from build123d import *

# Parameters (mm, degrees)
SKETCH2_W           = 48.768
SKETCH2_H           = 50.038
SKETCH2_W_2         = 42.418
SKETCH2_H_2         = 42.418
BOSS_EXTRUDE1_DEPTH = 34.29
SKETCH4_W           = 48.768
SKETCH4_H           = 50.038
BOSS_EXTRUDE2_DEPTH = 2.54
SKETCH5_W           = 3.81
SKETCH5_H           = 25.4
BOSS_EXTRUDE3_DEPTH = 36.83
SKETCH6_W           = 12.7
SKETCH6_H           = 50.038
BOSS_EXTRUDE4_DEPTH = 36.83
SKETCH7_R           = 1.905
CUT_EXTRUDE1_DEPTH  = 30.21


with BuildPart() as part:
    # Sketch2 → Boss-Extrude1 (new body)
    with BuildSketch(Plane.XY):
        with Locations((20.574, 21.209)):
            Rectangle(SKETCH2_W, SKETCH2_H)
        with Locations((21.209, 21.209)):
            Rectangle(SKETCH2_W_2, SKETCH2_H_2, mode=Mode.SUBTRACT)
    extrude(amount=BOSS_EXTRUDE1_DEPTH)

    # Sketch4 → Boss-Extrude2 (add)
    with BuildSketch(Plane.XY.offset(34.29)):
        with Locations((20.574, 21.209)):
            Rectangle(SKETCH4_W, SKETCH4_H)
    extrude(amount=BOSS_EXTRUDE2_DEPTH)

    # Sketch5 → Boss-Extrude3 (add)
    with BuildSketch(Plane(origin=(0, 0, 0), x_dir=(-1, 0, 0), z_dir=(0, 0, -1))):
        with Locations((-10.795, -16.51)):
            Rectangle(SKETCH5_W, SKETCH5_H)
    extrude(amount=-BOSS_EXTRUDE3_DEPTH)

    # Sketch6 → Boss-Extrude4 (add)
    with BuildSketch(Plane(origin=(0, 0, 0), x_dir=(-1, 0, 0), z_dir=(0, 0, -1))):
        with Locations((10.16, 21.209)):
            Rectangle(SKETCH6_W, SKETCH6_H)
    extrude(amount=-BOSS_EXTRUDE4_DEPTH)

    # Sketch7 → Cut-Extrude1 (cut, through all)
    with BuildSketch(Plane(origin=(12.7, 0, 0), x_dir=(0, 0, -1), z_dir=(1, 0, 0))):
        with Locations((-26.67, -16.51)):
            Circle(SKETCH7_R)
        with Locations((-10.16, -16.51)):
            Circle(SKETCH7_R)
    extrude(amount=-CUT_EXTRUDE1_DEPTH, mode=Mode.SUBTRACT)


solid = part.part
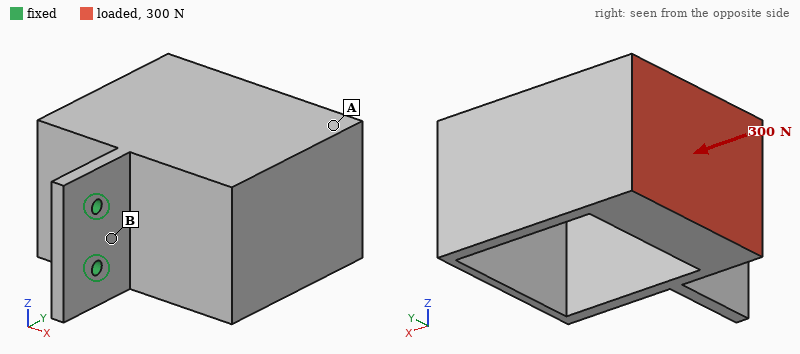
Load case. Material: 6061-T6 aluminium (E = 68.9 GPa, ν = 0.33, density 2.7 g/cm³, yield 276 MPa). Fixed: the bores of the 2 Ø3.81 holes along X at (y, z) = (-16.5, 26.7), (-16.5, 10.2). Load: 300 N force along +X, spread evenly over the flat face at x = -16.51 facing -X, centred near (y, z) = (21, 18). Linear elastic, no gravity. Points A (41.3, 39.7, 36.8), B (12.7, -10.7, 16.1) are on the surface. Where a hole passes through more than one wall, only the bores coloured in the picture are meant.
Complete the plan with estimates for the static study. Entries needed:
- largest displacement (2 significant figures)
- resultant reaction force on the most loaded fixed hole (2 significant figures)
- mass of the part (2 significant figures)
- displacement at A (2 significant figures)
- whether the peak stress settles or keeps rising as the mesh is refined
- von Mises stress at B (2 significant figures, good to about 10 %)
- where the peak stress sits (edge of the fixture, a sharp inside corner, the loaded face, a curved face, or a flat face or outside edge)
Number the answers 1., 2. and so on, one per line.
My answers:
1. 0.78 mm
2. 150 N
3. 150 g
4. 0.69 mm
5. keeps rising
6. 91 MPa
7. edge of the fixture
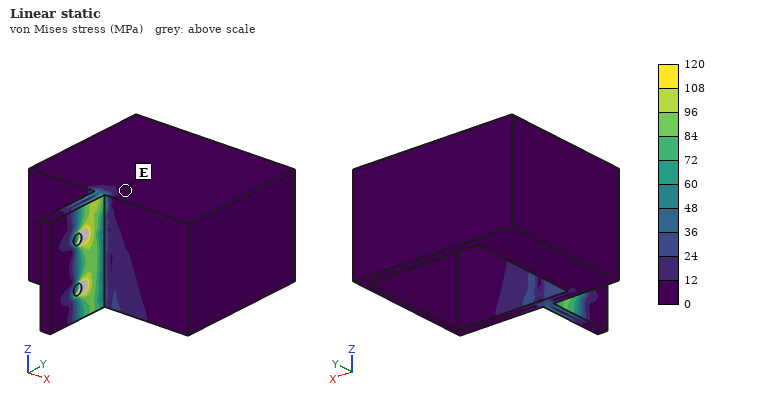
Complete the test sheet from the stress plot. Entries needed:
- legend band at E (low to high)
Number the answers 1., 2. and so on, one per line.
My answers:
1. 0 to 12 MPa
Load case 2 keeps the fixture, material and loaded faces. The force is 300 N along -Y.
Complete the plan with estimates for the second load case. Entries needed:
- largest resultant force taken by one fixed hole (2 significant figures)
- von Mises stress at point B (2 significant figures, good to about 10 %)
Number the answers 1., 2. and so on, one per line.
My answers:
1. 150 N
2. 77 MPa
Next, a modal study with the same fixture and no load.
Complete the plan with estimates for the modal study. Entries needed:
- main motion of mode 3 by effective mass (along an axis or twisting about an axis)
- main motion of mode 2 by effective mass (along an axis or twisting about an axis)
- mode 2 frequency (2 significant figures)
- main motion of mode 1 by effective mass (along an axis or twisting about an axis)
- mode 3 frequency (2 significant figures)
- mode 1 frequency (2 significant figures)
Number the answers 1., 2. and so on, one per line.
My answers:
1. along Z
2. twisting about Y
3. 1200 Hz
4. along X
5. 1300 Hz
6. 290 Hz
